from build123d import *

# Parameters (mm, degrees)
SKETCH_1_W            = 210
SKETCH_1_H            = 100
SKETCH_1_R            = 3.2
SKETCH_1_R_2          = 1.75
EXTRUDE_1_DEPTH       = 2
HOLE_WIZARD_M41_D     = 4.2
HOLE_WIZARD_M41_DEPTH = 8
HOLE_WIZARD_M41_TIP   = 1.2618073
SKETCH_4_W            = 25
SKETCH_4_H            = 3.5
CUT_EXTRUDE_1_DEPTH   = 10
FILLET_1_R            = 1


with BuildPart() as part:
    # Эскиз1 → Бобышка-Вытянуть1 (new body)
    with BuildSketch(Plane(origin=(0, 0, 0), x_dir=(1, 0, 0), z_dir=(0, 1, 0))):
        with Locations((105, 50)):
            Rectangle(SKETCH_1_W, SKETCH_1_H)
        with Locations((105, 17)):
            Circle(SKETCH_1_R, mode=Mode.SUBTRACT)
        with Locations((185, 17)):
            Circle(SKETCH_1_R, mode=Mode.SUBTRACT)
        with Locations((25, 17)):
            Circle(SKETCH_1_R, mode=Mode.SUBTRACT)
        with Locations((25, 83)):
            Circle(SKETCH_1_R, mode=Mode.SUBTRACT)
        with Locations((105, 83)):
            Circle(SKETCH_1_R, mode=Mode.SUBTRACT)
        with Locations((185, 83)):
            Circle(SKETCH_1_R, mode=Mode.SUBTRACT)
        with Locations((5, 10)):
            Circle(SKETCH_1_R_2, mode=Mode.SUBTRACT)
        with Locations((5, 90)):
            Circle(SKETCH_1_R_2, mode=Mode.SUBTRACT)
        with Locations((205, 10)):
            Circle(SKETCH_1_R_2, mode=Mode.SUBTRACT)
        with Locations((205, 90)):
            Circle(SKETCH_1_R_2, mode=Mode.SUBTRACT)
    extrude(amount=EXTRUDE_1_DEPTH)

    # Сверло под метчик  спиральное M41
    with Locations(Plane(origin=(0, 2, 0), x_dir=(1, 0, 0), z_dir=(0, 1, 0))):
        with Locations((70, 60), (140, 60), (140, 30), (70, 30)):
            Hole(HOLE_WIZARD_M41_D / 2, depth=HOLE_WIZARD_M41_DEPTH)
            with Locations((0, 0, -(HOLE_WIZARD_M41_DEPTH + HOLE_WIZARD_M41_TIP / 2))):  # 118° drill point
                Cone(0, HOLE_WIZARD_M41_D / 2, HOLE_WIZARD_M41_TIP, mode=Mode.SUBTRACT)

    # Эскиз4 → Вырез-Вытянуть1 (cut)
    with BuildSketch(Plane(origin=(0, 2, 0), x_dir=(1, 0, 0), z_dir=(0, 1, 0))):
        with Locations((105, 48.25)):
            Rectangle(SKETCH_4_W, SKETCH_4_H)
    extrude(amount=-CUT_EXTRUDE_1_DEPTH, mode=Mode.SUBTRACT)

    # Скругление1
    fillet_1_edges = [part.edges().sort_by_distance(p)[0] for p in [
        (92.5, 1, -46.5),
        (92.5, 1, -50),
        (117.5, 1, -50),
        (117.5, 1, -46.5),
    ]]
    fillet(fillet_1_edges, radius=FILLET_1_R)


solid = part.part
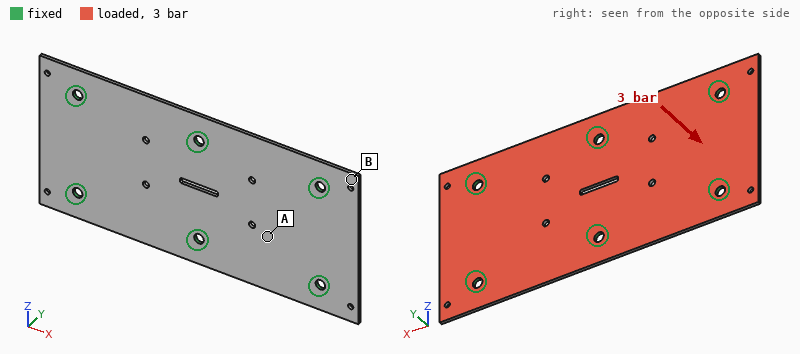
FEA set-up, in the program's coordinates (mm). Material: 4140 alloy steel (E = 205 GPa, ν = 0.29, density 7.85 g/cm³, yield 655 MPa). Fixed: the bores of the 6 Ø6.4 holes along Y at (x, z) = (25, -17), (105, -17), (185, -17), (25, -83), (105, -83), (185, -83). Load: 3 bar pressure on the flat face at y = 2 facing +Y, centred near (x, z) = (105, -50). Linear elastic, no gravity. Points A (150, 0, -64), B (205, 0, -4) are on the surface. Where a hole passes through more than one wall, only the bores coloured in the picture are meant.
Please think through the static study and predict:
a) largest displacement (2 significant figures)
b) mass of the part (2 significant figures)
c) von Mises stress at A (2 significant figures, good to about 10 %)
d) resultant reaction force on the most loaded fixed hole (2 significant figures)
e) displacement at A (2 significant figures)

0.32 mm
320 g
93 MPa
1.2 kN
0.29 mm
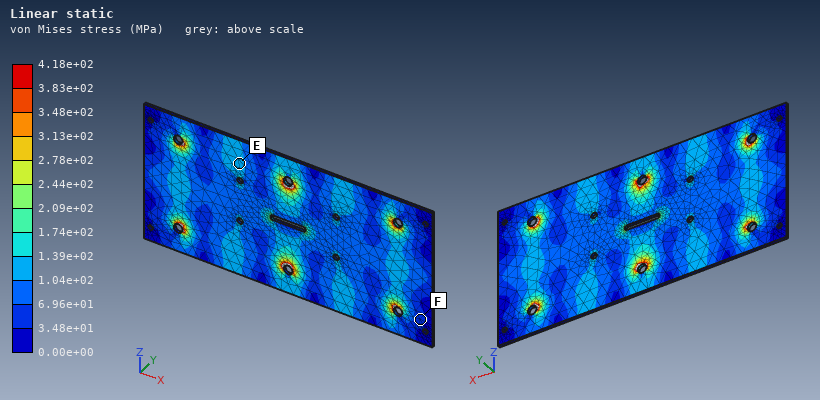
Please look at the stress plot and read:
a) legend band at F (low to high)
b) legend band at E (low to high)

3.48e+01 to 6.96e+01 MPa
1.04e+02 to 1.39e+02 MPa
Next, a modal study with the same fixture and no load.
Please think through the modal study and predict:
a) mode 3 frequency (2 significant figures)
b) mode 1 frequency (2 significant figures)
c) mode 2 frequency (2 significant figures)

1800 Hz
1400 Hz
1500 Hz
